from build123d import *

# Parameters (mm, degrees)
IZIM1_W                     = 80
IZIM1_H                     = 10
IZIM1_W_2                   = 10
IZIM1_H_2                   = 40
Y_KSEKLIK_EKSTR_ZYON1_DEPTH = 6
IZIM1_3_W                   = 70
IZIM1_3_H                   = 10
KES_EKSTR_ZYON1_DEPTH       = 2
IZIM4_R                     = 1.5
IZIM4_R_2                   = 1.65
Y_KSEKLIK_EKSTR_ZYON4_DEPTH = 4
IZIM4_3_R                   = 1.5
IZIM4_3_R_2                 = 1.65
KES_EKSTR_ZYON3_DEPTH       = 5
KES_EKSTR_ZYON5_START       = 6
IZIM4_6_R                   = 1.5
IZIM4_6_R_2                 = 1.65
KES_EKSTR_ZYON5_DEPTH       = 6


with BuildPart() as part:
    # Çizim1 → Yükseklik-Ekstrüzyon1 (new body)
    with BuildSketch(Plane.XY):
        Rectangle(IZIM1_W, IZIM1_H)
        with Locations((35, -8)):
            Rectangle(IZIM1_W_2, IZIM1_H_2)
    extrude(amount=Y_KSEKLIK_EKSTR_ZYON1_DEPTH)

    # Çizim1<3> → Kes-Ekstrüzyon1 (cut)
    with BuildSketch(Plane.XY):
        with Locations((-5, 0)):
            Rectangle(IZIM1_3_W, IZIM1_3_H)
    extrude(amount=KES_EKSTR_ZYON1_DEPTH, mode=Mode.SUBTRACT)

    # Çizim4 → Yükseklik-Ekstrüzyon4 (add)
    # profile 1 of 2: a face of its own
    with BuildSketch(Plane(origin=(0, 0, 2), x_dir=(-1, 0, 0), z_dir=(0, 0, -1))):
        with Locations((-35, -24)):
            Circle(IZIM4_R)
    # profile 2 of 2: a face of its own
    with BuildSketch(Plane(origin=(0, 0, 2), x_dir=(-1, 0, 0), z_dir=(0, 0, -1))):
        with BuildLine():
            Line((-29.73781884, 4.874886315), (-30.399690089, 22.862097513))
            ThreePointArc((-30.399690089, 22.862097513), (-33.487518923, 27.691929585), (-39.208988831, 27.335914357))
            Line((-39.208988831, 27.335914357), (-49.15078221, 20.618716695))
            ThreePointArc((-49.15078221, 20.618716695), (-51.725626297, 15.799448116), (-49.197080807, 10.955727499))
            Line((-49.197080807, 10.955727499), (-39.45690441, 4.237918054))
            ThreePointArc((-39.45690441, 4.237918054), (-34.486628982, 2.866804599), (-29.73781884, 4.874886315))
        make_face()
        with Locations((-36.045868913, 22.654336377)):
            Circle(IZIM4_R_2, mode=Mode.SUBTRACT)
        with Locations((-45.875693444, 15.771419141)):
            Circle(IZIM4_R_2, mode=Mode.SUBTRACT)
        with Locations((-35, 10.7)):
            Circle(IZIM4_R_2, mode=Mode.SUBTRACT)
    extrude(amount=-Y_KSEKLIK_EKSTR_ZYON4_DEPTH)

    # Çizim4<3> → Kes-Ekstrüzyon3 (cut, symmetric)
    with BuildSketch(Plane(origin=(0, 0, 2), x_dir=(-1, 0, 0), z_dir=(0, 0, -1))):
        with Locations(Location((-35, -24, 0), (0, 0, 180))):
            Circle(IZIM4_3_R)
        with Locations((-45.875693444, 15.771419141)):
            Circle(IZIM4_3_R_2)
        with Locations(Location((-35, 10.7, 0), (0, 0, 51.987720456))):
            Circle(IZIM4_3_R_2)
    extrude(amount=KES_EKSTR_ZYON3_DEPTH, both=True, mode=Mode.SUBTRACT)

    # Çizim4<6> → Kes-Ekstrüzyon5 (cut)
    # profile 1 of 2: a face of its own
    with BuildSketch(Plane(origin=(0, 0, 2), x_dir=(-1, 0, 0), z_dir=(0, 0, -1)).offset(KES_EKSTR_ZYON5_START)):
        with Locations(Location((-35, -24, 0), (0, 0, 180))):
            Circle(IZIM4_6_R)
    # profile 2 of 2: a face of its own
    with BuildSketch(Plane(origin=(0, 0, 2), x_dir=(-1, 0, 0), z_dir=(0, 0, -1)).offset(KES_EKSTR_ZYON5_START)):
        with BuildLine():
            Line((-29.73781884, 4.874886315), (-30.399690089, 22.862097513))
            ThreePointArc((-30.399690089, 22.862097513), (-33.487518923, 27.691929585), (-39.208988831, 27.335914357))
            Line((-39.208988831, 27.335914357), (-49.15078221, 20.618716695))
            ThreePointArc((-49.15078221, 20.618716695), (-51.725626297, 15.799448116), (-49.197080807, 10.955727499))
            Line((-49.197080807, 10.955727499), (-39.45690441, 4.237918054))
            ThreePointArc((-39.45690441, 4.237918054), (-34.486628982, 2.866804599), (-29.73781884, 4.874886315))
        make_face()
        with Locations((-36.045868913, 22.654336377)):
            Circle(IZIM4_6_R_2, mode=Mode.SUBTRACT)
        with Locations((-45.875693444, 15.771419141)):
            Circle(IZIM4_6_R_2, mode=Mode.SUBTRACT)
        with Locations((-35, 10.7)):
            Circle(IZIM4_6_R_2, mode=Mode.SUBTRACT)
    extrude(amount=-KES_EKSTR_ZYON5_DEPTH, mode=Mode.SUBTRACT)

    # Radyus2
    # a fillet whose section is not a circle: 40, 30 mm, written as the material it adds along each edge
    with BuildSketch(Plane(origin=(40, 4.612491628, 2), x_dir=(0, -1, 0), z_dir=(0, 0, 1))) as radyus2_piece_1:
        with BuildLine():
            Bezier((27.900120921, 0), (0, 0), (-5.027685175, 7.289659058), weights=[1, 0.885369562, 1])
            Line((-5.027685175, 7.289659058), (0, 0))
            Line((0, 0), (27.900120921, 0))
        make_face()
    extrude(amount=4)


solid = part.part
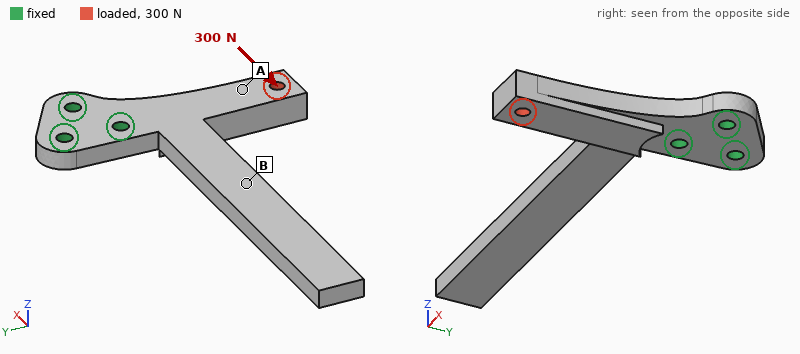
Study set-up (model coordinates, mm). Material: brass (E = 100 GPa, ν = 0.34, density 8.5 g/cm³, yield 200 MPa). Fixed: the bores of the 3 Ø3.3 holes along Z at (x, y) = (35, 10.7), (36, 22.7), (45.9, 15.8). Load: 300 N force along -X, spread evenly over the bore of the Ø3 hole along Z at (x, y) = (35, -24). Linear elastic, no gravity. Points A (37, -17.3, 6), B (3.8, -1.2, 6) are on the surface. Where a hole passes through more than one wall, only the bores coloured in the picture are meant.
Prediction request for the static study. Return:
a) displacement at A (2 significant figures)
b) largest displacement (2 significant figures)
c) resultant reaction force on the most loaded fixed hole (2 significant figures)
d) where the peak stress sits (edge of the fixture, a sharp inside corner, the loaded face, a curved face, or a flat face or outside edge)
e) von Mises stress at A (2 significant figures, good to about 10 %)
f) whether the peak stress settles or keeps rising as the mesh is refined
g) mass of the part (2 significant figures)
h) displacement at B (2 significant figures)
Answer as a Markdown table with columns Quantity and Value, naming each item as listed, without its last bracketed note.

| Quantity | Value |
|---|---|
| displacement at A | 41 µm |
| largest displacement | 92 µm |
| resultant reaction force on the most loaded fixed hole | 770 N |
| where the peak stress sits | edge of the fixture |
| von Mises stress at A | 14 MPa |
| whether the peak stress settles or keeps rising as the mesh is refined | keeps rising |
| mass of the part | 53 g |
| displacement at B | 40 µm |
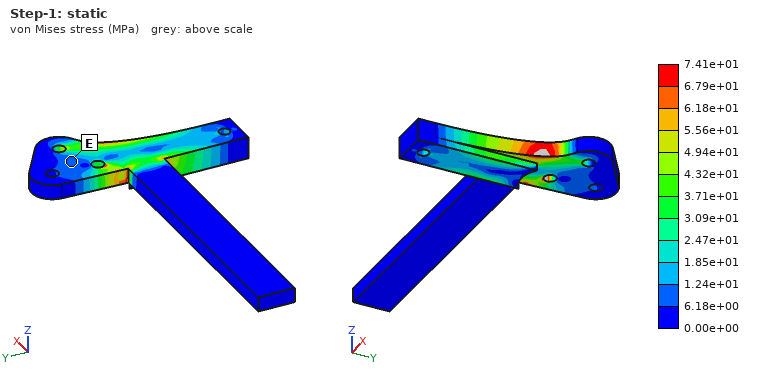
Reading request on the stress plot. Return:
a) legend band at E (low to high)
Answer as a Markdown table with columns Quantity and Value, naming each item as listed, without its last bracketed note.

| Quantity | Value |
|---|---|
| legend band at E | 6.18e+00 to 1.24e+01 MPa |
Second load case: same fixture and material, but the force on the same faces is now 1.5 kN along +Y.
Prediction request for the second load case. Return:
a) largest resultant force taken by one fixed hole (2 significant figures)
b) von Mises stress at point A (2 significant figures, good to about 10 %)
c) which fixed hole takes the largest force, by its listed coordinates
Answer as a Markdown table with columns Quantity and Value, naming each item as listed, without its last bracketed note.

| Quantity | Value |
|---|---|
| largest resultant force taken by one fixed hole | 1.3 kN |
| von Mises stress at point A | 25 MPa |
| which fixed hole takes the largest force, by its listed coordinates | (35, 10.7) |
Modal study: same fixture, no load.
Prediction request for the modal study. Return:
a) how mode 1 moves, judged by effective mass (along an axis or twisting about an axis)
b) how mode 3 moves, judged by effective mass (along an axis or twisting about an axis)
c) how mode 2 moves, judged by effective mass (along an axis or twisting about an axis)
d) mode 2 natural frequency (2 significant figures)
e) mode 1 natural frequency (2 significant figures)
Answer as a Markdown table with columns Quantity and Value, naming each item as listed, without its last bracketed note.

| Quantity | Value |
|---|---|
| how mode 1 moves, judged by effective mass | along Z |
| how mode 3 moves, judged by effective mass | along Z |
| how mode 2 moves, judged by effective mass | along Y |
| mode 2 natural frequency | 920 Hz |
| mode 1 natural frequency | 380 Hz |
